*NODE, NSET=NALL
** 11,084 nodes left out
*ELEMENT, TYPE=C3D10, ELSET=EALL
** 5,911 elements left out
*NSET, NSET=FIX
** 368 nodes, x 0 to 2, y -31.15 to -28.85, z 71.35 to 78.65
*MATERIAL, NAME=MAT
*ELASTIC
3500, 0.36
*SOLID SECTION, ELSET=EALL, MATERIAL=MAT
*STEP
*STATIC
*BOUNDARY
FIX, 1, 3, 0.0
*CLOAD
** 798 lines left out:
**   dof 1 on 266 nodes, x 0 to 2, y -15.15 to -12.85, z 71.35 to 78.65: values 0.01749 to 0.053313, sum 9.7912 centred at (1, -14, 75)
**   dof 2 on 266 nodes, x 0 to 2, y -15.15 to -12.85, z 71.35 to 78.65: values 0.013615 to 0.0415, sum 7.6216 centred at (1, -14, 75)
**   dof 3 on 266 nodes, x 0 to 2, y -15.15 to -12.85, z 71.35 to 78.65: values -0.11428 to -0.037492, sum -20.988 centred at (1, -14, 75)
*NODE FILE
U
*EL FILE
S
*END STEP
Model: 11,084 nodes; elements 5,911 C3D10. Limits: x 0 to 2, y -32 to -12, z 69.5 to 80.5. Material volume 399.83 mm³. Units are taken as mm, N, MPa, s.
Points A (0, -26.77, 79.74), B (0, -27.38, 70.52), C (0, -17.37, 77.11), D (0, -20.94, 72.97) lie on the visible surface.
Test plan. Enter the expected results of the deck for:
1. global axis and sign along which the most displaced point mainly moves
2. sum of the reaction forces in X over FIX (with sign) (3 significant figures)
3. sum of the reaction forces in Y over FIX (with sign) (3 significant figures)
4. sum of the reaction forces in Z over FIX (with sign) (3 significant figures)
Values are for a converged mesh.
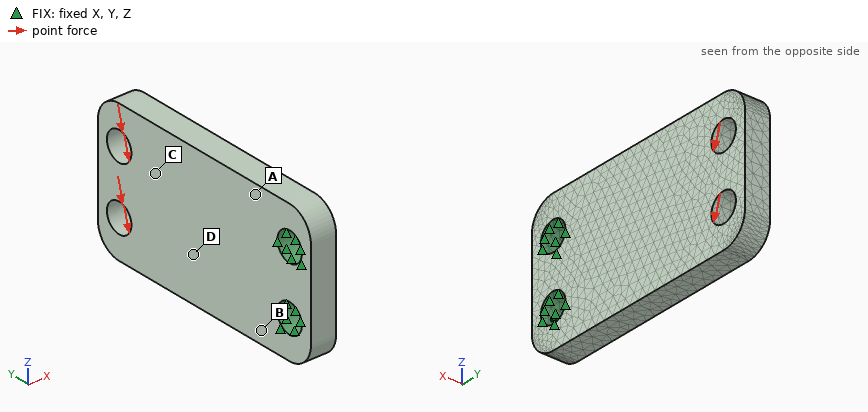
+X
-9.79 N
-7.62 N
21.0 N
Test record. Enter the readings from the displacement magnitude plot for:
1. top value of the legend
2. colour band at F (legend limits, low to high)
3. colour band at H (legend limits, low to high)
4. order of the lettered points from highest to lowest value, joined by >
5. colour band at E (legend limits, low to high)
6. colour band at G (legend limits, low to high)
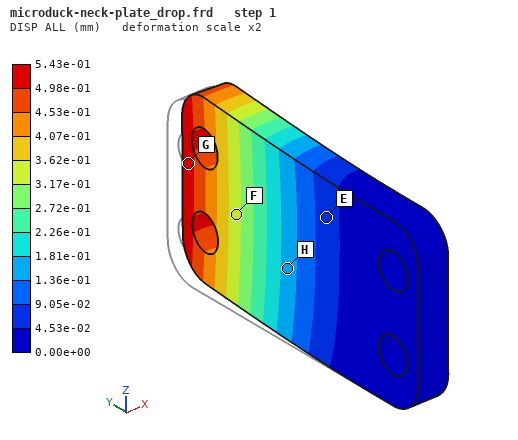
5.43e-01 mm
3.17e-01 to 3.62e-01 mm
1.36e-01 to 1.81e-01 mm
G > F > H > E
4.53e-02 to 9.05e-02 mm
4.98e-01 to 5.43e-01 mm
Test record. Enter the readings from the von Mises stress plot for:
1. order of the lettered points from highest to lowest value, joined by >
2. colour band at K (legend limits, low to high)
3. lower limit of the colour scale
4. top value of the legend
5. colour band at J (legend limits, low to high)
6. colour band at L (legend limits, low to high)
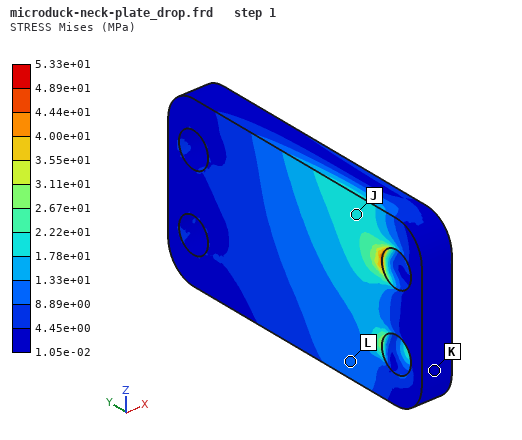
J > L > K
1.05e-02 to 4.45e+00 MPa
1.05e-02 MPa
5.33e+01 MPa
1.78e+01 to 2.22e+01 MPa
8.89e+00 to 1.33e+01 MPa
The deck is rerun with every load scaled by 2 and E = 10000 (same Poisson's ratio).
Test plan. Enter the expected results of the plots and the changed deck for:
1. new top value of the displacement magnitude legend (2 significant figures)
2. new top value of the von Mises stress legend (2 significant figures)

0.38 mm
110 MPa
